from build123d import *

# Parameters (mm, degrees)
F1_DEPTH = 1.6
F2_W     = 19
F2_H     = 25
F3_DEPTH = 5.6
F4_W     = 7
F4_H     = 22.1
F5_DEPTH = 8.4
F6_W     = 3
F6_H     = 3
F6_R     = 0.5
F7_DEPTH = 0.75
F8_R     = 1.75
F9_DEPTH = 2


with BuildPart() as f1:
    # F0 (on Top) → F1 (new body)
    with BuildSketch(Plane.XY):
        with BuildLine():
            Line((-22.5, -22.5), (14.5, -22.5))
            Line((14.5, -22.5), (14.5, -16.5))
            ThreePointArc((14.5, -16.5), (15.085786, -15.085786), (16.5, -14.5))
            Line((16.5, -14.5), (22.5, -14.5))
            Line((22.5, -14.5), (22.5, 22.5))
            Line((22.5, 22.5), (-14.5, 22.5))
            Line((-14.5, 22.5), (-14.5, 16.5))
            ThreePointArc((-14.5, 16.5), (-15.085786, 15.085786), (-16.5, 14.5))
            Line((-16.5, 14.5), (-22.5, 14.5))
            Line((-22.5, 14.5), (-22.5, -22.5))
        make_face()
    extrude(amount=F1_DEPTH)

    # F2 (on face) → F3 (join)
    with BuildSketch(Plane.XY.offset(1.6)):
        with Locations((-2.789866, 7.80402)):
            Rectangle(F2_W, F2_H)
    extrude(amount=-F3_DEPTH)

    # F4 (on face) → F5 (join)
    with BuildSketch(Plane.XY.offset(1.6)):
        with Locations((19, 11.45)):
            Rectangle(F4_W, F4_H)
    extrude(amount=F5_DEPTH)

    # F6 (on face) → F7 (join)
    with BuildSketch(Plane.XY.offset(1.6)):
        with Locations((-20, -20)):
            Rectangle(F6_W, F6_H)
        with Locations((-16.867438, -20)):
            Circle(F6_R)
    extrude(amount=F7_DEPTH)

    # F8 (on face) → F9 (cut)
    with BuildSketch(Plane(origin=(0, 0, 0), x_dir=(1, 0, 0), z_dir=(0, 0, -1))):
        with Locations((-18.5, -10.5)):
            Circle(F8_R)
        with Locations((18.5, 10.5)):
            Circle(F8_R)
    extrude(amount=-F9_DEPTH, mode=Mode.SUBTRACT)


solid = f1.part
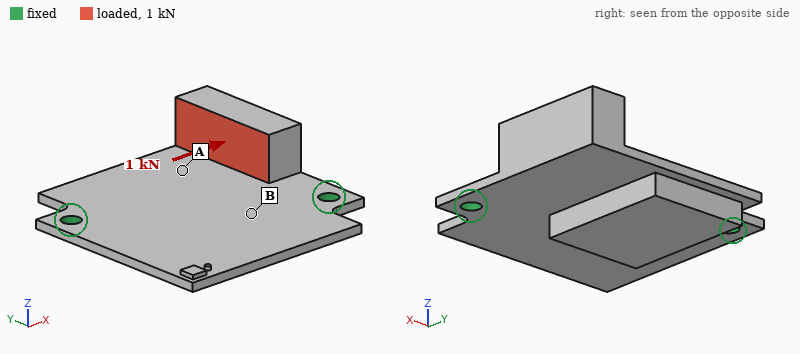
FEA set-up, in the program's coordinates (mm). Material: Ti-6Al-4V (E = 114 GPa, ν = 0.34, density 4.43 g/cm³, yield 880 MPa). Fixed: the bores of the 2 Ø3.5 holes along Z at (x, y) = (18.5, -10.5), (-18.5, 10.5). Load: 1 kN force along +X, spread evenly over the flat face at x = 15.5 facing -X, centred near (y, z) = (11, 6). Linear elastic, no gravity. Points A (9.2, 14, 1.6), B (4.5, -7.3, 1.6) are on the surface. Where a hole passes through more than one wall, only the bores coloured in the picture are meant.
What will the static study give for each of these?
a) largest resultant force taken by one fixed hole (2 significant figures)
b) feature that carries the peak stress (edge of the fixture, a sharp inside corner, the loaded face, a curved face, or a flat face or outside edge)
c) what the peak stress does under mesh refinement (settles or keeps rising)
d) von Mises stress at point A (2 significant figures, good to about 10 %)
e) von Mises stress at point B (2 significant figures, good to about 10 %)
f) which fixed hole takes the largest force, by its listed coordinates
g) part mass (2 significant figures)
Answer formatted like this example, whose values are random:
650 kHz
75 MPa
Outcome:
670 N
edge of the fixture
keeps rising
230 MPa
59 MPa
(-18.5, 10.5)
28 g
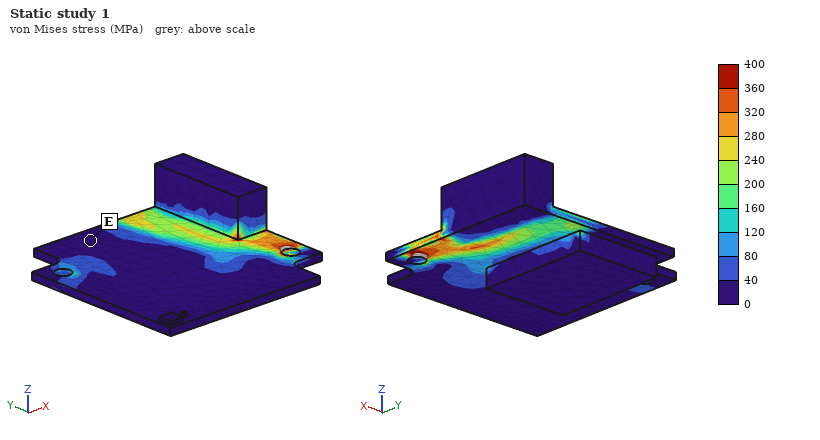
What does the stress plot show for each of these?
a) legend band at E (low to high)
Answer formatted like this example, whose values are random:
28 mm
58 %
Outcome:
0 to 40 MPa
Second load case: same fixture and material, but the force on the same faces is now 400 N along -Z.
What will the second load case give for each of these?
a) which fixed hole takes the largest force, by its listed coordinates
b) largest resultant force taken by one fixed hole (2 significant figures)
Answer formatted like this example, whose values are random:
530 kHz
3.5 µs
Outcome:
(18.5, -10.5)
360 N
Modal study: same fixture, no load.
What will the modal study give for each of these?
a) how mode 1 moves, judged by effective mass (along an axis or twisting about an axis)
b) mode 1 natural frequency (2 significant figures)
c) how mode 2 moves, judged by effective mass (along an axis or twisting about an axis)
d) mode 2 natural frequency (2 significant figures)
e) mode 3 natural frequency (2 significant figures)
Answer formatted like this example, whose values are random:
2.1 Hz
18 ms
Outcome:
along Z
1200 Hz
along Z
2800 Hz
3900 Hz
